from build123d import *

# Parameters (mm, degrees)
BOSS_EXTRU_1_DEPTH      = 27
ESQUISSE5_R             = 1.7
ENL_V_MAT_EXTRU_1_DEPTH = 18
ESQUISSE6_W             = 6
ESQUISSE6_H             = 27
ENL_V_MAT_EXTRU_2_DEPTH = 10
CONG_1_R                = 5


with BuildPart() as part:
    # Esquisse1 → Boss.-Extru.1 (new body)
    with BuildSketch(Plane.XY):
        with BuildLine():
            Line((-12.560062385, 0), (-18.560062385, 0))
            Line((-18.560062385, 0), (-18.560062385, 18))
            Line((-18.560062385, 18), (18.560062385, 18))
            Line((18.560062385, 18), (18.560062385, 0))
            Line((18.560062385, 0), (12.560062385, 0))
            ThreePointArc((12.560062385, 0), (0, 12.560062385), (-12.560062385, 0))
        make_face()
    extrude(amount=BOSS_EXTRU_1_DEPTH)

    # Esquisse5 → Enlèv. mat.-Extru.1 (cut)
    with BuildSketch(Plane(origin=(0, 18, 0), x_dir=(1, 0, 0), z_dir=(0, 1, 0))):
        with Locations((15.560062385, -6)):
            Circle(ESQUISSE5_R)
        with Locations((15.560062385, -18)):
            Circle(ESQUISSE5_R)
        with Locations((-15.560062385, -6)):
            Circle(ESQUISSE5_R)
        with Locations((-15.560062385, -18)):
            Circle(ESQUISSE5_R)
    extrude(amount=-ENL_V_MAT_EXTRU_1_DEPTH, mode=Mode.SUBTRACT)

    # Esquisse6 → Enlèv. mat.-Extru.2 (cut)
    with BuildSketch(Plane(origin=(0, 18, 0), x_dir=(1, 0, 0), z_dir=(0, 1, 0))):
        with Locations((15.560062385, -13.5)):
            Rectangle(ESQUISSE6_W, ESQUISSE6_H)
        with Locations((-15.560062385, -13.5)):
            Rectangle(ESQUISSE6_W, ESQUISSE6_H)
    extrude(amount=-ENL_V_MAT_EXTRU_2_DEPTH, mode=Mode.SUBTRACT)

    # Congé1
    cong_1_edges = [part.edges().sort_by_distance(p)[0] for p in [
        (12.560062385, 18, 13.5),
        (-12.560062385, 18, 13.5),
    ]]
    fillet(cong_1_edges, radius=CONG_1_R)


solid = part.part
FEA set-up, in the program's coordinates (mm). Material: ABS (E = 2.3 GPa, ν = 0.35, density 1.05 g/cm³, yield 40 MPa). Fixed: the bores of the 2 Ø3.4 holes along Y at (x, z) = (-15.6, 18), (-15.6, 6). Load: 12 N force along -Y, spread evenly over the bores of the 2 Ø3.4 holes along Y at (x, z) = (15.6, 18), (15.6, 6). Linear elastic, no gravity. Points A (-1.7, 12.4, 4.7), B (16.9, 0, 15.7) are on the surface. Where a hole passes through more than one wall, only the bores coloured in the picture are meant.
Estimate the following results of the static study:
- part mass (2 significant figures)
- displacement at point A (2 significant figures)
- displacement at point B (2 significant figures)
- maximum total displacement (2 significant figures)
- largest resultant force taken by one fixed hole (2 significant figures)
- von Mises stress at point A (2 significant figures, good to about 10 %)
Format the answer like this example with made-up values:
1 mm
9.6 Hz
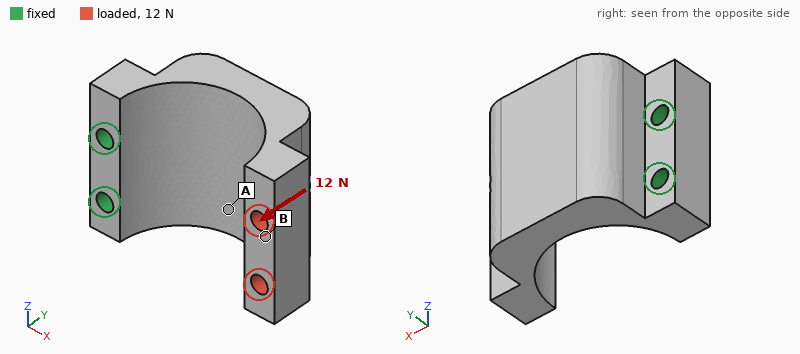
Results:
7.9 g
0.16 mm
0.49 mm
0.52 mm
6.8 N
1.6 MPa
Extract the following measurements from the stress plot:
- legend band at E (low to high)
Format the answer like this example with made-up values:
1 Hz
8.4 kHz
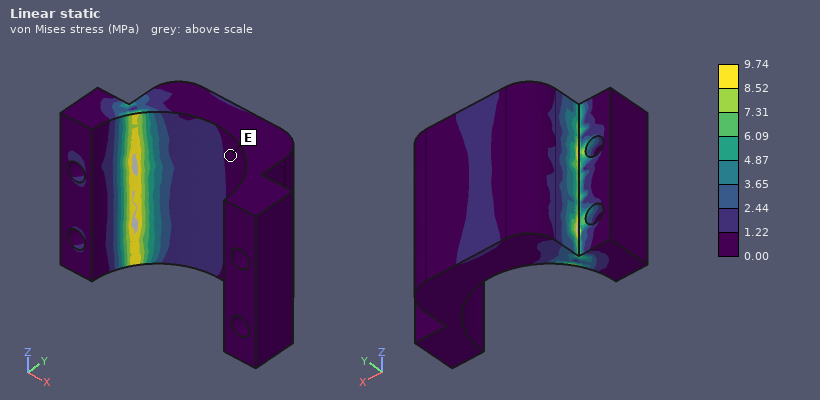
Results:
0.00 to 1.22 MPa
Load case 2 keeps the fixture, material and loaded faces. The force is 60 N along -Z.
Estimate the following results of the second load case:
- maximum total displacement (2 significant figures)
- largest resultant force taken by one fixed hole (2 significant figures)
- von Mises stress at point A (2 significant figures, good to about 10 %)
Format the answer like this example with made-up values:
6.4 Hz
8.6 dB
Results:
0.55 mm
120 N
6.9 MPa
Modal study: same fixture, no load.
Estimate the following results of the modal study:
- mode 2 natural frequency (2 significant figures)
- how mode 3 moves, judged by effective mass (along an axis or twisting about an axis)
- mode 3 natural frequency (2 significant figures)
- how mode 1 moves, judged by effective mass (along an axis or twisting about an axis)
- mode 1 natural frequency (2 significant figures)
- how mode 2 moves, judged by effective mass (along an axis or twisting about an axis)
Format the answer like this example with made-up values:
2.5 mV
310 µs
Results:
1200 Hz
along X
2300 Hz
along Y
490 Hz
along Z
